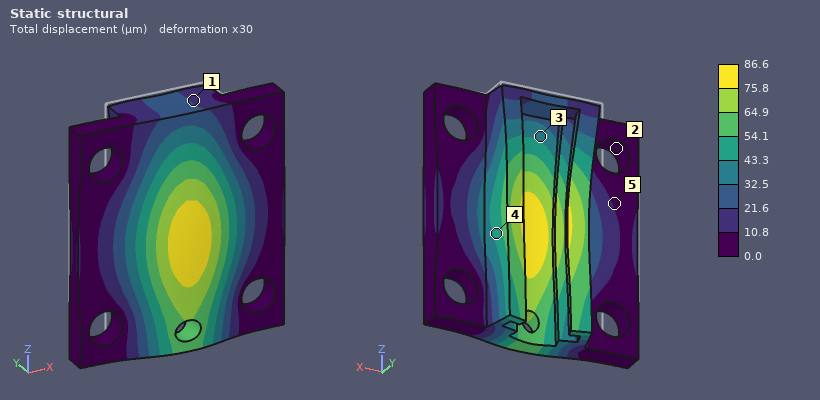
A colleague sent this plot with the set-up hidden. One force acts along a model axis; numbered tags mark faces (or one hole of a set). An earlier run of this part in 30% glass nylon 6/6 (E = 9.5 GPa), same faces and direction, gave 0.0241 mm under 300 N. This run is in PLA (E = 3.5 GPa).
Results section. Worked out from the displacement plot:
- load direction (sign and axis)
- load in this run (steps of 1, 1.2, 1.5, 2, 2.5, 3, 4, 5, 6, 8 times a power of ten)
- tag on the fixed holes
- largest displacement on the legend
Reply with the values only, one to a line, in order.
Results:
-Y
400 N
2
86.6 µm
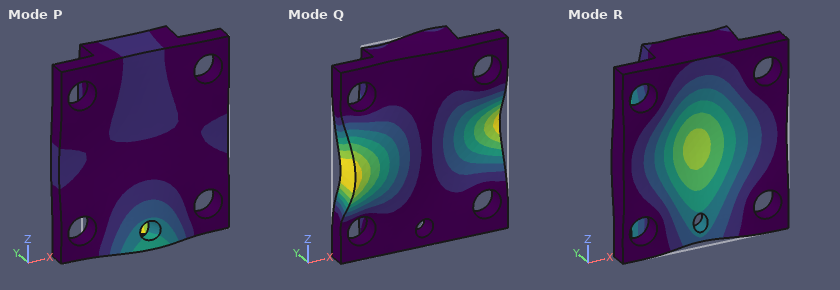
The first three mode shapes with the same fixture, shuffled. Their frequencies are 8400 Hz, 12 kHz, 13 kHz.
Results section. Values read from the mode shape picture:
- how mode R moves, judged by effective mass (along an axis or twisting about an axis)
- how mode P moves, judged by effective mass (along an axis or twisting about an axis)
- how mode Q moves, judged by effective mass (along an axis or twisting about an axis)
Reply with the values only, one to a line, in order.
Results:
along Y
twisting about X
twisting about Z
